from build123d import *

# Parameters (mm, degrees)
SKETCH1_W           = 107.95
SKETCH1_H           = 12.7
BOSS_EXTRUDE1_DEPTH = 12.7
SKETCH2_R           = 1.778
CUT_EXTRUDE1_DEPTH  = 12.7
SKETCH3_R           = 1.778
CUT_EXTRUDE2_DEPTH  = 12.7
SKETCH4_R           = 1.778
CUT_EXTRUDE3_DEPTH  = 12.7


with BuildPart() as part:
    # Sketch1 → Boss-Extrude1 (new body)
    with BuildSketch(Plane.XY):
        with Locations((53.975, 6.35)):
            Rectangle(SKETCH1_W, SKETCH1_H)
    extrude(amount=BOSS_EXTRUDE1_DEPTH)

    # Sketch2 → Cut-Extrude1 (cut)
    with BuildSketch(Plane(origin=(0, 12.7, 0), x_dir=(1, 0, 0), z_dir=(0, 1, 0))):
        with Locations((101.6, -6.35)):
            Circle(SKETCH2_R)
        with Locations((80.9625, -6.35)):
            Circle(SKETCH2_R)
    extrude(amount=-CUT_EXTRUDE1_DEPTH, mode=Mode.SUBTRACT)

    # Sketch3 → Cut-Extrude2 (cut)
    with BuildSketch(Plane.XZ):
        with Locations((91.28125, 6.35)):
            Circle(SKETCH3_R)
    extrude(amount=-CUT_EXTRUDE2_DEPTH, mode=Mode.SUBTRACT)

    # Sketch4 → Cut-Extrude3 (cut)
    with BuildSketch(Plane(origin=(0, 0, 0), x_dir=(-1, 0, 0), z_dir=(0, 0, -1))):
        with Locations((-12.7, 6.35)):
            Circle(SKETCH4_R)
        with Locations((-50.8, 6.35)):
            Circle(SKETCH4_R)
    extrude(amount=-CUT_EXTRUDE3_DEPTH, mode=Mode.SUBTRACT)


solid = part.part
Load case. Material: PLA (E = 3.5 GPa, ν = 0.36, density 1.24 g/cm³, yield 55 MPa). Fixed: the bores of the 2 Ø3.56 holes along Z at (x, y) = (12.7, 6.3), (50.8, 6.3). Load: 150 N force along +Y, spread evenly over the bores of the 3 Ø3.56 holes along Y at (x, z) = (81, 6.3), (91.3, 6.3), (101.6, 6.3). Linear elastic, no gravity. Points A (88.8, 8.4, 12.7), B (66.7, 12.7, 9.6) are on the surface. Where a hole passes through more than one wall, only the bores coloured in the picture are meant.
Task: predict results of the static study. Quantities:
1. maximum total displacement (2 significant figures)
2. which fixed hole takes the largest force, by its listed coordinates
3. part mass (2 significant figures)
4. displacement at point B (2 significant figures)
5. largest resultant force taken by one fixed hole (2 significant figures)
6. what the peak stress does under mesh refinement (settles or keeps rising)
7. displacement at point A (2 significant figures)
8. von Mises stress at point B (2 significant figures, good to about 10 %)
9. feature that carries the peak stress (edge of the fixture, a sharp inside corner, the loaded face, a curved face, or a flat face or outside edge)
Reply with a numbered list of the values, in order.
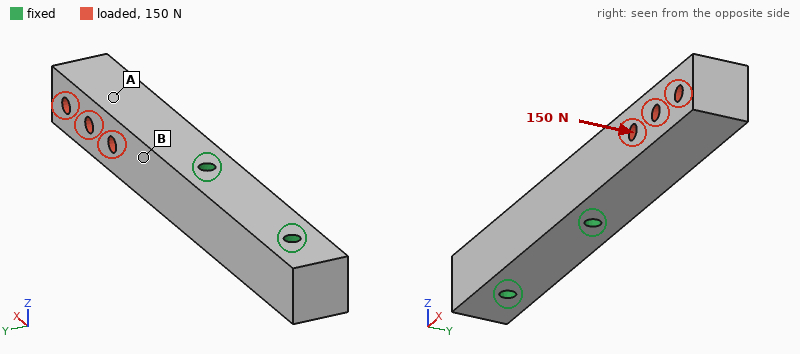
1. 1.0 mm
2. (50.8, 6.3)
3. 21 g
4. 0.19 mm
5. 230 N
6. keeps rising
7. 0.59 mm
8. 11 MPa
9. edge of the fixture
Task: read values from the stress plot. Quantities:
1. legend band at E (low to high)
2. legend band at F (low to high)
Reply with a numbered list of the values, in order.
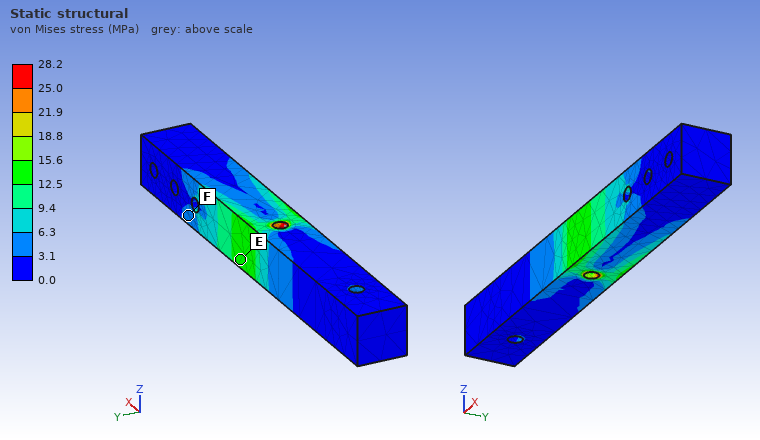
1. 12.5 to 15.6 MPa
2. 3.1 to 6.3 MPa
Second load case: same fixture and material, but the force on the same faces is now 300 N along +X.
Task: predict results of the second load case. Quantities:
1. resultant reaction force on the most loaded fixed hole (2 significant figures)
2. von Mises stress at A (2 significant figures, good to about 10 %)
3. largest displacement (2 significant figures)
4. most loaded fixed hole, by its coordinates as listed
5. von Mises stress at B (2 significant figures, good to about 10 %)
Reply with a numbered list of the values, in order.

1. 290 N
2. 1.3 MPa
3. 25 µm
4. (50.8, 6.3)
5. 1.9 MPa
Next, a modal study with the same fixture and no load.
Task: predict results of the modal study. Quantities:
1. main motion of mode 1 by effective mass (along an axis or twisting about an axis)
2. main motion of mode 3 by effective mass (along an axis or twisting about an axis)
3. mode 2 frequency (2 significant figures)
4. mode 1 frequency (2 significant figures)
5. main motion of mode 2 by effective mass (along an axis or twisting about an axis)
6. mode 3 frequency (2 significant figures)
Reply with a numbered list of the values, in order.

1. along Y
2. twisting about X
3. 1000 Hz
4. 900 Hz
5. along Z
6. 4100 Hz
